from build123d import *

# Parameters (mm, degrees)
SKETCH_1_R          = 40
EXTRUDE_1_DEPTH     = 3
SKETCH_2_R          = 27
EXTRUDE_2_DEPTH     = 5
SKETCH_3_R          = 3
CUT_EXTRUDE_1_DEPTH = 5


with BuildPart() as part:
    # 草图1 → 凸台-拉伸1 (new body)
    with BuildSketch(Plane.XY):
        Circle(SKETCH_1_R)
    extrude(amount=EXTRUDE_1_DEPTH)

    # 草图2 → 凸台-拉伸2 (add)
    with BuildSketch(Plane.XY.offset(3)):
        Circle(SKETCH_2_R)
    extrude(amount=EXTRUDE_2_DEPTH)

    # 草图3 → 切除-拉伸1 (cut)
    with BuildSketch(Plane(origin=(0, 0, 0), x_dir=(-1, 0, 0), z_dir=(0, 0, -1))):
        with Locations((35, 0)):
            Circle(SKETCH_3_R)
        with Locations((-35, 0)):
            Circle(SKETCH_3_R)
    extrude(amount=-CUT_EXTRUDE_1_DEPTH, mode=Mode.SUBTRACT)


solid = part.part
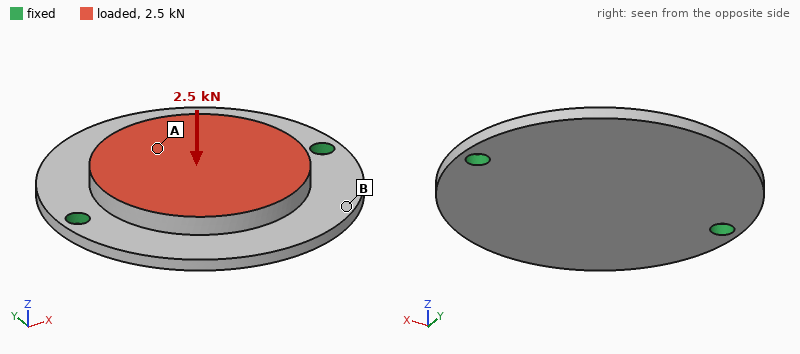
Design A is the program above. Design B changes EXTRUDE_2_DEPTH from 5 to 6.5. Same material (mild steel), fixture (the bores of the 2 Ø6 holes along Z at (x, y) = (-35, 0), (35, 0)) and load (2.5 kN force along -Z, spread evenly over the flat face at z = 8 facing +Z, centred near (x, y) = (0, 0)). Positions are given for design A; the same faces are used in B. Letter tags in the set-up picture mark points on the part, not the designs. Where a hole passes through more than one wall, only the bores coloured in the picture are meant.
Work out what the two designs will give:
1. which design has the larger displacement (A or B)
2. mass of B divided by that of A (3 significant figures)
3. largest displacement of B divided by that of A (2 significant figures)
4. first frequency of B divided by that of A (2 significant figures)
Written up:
A
1.13
0.72
0.98
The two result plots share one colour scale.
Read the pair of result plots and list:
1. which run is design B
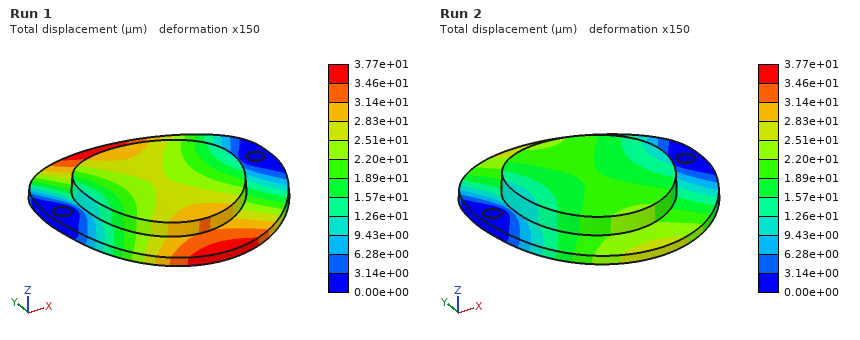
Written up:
Run 2
